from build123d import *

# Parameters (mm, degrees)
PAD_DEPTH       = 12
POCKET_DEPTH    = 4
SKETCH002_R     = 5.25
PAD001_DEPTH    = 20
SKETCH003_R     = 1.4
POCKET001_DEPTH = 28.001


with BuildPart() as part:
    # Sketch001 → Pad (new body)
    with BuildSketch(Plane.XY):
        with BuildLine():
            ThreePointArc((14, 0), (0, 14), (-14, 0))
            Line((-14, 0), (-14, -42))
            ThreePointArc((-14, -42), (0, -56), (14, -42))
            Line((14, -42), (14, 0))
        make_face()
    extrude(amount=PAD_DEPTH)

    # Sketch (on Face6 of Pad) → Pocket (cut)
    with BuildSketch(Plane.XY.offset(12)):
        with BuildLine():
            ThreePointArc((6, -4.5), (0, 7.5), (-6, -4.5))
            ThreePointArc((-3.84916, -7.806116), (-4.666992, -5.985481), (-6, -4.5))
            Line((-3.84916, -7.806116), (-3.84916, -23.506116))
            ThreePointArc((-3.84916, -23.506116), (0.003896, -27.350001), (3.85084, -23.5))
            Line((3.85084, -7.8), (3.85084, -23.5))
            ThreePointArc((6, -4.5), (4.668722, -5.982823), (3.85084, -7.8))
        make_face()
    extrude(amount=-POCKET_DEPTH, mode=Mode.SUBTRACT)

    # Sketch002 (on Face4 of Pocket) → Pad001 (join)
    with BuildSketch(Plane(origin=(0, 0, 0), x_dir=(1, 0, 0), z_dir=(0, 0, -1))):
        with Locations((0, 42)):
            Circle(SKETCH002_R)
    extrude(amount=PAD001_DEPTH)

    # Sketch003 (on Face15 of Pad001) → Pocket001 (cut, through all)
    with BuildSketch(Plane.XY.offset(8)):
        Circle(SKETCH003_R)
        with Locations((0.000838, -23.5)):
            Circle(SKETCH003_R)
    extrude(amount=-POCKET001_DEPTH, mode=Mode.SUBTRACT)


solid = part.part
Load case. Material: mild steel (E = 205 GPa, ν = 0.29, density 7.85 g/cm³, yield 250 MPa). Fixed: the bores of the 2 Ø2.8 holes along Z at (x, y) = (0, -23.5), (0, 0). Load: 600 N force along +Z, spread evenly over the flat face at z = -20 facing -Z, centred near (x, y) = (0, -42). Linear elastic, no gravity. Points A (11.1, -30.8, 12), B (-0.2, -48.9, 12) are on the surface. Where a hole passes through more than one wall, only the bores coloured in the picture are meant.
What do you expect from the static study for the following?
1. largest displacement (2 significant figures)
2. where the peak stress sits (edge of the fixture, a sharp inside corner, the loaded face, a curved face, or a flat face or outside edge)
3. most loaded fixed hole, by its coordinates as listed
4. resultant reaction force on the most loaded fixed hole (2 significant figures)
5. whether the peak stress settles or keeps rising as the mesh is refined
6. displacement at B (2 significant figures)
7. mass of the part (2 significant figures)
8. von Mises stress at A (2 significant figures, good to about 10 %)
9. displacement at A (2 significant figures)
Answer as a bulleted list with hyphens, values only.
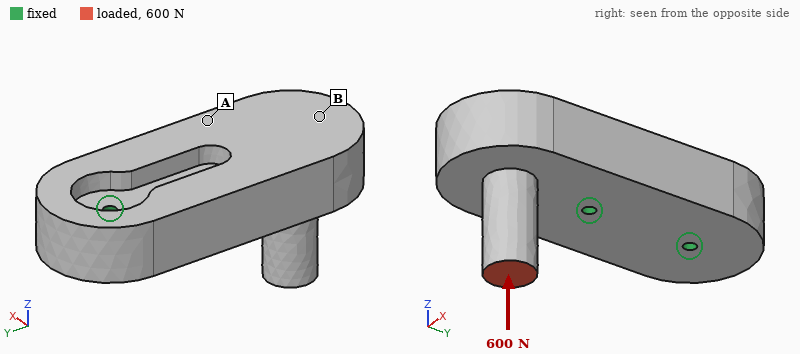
- 9.1 µm
- edge of the fixture
- (0, -23.5)
- 920 N
- keeps rising
- 6.4 µm
- 170 g
- 10 MPa
- 2.2 µm
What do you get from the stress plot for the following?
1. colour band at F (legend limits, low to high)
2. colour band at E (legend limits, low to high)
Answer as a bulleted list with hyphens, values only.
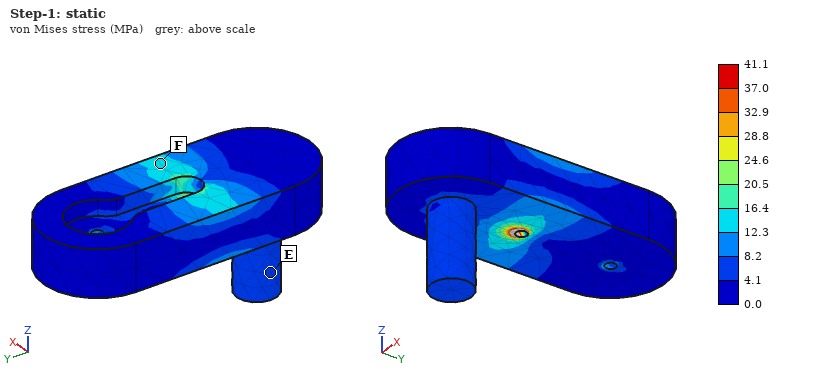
- 12.3 to 16.4 MPa
- 4.1 to 8.2 MPa
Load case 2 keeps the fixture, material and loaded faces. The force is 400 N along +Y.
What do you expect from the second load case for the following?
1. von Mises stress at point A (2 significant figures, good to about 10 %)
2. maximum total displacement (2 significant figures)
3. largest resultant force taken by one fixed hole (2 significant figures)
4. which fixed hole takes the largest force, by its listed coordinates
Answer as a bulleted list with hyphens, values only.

- 15 MPa
- 24 µm
- 550 N
- (0, -23.5)
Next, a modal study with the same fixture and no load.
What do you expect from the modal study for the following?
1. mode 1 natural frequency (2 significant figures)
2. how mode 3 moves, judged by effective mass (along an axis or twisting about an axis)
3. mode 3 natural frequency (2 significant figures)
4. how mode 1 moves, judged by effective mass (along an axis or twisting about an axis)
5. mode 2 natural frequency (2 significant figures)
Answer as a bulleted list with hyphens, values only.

- 5800 Hz
- along X
- 9900 Hz
- along Z
- 7800 Hz
